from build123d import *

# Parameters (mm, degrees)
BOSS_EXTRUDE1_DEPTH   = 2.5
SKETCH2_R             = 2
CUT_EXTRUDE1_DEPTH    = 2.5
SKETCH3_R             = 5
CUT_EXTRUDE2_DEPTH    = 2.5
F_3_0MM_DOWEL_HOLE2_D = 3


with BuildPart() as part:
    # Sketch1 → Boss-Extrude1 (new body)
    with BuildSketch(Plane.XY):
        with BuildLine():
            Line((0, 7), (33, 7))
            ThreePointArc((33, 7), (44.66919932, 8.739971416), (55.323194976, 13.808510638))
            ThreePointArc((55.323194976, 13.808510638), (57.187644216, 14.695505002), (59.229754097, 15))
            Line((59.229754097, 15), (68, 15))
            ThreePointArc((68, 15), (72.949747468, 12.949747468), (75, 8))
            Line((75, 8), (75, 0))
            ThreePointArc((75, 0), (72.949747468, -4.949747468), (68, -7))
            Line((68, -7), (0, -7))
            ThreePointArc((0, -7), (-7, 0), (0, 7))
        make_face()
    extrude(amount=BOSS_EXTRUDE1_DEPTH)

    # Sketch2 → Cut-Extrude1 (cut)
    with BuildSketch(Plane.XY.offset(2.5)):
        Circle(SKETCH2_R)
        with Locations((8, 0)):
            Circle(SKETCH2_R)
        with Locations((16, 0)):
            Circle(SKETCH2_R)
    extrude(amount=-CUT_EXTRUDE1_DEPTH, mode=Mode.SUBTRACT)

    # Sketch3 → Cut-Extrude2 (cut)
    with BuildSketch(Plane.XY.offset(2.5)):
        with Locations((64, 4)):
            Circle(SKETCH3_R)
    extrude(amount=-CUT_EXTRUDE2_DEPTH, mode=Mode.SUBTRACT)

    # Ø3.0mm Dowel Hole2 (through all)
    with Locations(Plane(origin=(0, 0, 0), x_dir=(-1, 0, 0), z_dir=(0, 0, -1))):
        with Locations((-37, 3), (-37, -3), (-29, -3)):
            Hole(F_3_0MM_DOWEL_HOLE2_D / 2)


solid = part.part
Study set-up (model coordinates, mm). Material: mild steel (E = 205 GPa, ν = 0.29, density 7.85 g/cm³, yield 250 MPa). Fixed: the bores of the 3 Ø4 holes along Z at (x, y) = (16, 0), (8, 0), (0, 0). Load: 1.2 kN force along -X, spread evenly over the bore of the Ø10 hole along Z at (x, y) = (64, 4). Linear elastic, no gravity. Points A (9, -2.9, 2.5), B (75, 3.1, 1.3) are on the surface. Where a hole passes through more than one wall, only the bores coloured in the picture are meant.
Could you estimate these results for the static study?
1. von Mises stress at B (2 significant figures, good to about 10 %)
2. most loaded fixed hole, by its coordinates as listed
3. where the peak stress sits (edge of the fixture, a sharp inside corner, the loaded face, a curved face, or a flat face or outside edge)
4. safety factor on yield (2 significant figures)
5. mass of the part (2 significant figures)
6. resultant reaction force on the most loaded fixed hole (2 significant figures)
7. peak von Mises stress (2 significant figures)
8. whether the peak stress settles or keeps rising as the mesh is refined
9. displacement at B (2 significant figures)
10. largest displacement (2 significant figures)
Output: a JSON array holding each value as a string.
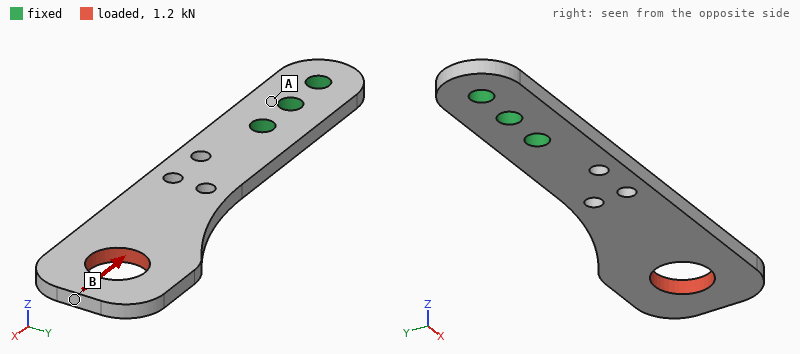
["35 MPa", "(16, 0)", "a curved face", "1.2", "23 g", "1.0 kN", "210 MPa", "settles", "69 µm", "71 µm"]
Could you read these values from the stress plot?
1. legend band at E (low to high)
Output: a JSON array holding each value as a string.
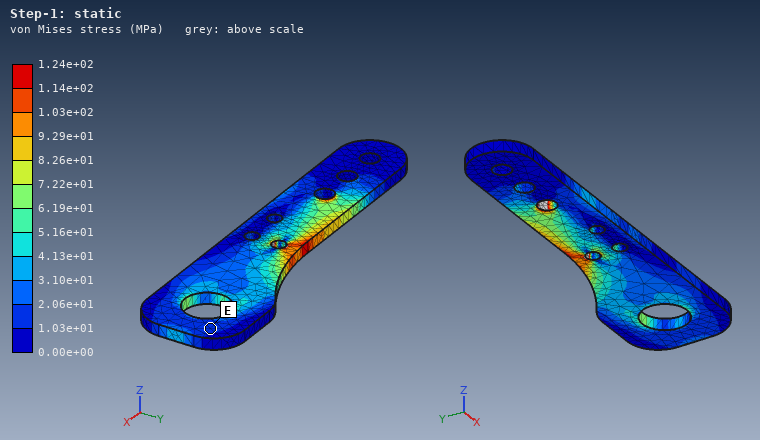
["1.03e+01 to 2.06e+01 MPa"]
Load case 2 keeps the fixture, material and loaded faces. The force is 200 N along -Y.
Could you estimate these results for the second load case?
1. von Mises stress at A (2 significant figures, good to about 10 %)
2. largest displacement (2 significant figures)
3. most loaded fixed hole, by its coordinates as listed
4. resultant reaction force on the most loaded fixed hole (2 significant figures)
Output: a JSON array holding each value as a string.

["30 MPa", "0.11 mm", "(16, 0)", "680 N"]
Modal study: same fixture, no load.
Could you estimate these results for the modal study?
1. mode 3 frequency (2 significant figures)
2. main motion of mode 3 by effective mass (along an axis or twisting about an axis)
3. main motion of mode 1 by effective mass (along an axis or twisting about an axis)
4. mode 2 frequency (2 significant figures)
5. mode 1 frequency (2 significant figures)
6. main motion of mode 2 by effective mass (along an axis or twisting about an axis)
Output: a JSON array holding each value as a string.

["2800 Hz", "twisting about X", "along Z", "2500 Hz", "540 Hz", "along Y"]
